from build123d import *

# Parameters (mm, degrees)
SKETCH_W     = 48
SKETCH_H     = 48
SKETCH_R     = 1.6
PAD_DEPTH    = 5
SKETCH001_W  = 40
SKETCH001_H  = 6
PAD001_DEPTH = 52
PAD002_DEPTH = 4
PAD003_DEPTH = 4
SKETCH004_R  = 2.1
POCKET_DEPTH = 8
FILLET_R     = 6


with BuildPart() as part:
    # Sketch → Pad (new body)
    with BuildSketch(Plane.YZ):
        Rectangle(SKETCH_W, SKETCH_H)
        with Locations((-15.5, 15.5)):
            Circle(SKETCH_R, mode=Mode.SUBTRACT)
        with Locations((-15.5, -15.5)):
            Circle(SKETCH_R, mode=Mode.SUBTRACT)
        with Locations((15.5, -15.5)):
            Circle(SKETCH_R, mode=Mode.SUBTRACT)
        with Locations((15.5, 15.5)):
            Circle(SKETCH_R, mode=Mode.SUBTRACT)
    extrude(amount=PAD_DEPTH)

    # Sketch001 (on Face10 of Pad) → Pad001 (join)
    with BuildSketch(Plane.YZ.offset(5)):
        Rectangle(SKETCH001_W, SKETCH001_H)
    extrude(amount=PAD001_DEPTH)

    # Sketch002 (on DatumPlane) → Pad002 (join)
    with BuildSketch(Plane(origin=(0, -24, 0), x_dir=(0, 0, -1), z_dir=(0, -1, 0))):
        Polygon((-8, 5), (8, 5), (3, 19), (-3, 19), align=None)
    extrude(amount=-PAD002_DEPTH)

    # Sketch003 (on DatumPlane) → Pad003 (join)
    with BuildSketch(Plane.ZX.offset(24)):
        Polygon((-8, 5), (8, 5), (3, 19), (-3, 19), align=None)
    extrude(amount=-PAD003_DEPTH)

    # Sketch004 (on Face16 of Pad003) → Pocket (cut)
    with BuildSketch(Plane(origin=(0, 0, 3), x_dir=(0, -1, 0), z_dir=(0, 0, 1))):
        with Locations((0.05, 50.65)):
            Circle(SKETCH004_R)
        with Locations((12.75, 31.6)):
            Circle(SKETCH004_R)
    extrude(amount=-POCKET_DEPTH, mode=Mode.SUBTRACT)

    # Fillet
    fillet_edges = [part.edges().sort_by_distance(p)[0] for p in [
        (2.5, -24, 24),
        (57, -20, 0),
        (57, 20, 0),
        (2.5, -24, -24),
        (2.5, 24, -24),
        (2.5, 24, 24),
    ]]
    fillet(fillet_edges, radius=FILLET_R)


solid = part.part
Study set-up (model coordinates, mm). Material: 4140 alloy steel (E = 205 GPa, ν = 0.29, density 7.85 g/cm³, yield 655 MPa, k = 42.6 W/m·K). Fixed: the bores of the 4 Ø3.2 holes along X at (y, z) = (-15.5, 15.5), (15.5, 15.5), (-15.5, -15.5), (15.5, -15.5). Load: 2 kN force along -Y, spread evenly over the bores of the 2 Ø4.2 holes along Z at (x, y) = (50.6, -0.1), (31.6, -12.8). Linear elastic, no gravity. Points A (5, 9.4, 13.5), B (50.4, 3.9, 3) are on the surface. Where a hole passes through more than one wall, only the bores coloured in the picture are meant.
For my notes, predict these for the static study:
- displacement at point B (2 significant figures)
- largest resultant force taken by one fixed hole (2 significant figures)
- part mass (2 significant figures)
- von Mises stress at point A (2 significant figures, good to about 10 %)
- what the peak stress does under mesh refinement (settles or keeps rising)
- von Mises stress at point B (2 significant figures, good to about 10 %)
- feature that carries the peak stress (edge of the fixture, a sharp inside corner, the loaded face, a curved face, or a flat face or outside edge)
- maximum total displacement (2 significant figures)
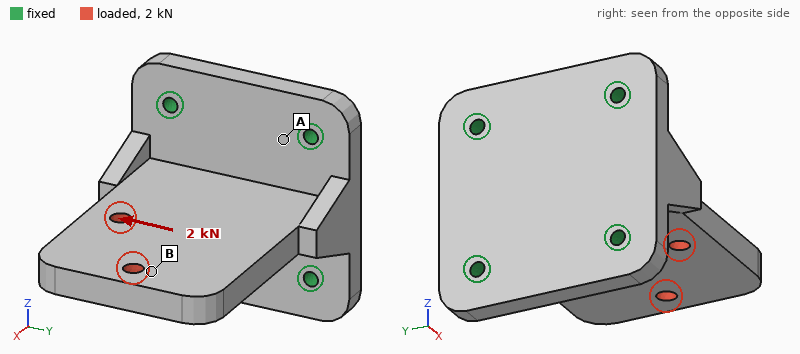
32 µm
1.3 kN
190 g
31 MPa
keeps rising
13 MPa
edge of the fixture
37 µm
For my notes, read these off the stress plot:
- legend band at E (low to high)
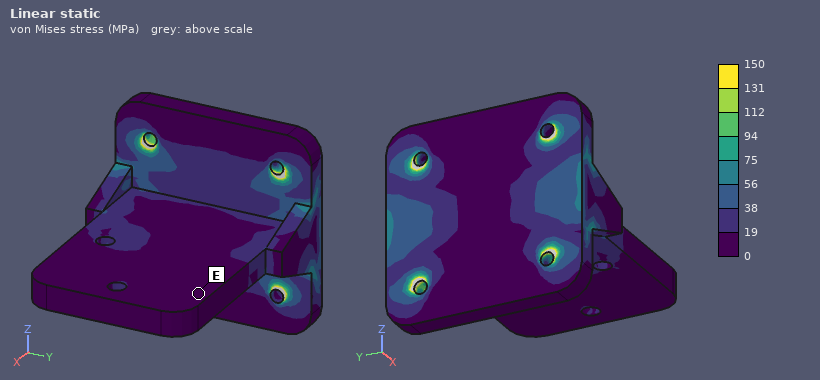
0 to 19 MPa
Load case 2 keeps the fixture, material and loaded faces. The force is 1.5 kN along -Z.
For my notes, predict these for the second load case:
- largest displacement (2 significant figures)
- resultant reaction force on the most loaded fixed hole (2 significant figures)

0.27 mm
1.4 kN
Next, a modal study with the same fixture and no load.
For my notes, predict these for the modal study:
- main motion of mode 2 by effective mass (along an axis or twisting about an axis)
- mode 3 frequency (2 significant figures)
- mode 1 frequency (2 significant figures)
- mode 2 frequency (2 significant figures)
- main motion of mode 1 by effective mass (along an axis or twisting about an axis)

along Y
5700 Hz
1900 Hz
5100 Hz
along Z
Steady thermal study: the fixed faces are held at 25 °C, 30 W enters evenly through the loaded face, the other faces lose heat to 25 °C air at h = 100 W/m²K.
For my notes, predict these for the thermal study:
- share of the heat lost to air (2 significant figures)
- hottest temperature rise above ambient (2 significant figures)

68 %
71 K
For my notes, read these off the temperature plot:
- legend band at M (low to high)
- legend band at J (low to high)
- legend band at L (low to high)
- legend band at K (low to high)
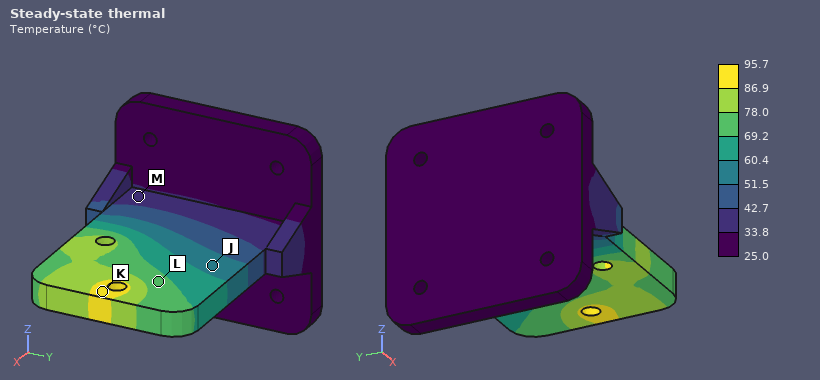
33.8 to 42.7 °C
51.5 to 60.4 °C
69.2 to 78.0 °C
86.9 to 95.7 °C
